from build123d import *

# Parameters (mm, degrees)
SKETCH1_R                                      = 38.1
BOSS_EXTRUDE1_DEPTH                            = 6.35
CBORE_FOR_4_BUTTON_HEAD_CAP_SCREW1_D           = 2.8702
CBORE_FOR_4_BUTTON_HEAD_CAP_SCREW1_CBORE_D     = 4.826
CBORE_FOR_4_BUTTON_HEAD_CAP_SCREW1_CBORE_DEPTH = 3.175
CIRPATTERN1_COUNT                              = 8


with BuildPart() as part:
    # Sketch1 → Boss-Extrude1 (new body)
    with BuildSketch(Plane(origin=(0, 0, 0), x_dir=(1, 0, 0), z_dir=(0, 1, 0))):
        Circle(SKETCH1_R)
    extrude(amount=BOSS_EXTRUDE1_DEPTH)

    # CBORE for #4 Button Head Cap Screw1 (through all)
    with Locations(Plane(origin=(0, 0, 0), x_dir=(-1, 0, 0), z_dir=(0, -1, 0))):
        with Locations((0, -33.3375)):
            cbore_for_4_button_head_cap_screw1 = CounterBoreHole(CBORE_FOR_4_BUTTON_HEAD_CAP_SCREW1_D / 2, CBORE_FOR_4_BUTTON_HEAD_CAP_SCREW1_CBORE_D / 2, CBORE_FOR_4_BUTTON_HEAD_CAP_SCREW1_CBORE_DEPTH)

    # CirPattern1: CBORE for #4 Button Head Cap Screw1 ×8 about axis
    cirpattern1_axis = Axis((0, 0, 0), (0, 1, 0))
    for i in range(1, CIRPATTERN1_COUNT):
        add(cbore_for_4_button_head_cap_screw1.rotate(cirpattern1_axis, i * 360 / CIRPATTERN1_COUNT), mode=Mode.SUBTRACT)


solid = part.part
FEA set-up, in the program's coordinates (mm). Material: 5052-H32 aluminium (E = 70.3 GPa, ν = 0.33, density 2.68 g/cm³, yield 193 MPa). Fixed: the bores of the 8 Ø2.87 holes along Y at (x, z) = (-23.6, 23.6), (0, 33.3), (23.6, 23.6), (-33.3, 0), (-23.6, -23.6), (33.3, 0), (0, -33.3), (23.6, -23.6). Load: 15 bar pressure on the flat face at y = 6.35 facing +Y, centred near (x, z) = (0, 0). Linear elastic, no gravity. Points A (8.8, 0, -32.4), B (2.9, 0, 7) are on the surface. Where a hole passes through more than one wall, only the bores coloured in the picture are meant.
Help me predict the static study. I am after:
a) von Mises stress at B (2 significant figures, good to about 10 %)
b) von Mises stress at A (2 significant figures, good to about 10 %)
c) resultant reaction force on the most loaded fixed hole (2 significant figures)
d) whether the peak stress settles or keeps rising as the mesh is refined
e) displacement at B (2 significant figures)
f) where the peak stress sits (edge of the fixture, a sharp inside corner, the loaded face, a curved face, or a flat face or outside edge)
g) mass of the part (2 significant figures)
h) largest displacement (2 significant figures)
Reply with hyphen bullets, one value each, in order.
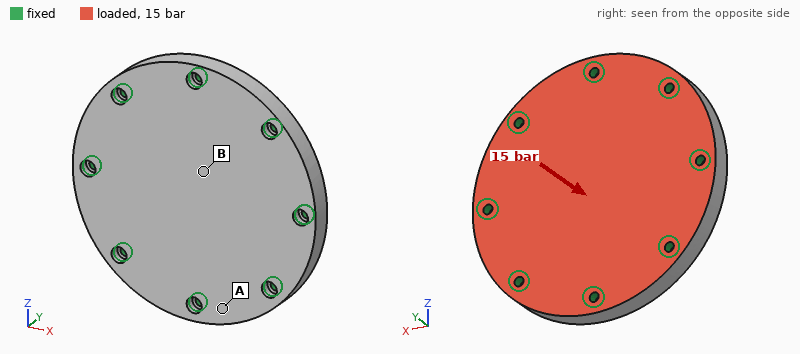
- 32 MPa
- 15 MPa
- 990 N
- keeps rising
- 36 µm
- edge of the fixture
- 76 g
- 39 µm
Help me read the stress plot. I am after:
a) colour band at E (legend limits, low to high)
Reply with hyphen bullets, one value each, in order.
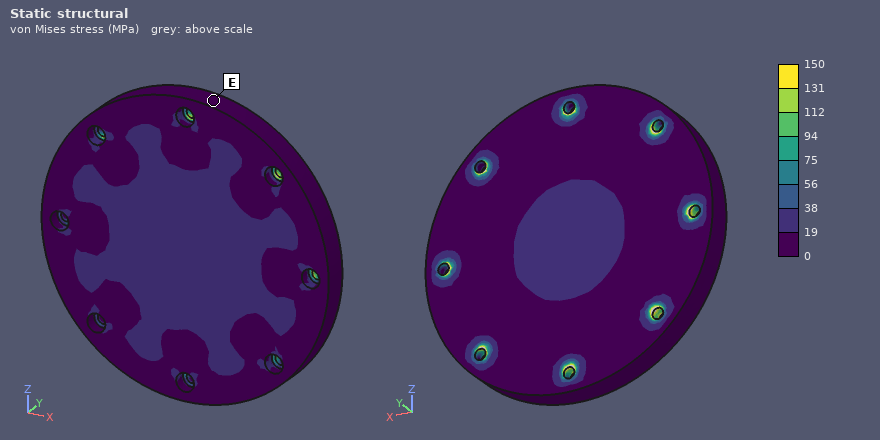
- 0 to 19 MPa
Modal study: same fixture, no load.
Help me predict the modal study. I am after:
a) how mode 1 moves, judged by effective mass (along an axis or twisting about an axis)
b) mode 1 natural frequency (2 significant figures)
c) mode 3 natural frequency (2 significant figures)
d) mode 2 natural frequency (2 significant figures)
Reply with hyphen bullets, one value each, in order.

- along Y
- 9200 Hz
- 19 kHz
- 19 kHz
